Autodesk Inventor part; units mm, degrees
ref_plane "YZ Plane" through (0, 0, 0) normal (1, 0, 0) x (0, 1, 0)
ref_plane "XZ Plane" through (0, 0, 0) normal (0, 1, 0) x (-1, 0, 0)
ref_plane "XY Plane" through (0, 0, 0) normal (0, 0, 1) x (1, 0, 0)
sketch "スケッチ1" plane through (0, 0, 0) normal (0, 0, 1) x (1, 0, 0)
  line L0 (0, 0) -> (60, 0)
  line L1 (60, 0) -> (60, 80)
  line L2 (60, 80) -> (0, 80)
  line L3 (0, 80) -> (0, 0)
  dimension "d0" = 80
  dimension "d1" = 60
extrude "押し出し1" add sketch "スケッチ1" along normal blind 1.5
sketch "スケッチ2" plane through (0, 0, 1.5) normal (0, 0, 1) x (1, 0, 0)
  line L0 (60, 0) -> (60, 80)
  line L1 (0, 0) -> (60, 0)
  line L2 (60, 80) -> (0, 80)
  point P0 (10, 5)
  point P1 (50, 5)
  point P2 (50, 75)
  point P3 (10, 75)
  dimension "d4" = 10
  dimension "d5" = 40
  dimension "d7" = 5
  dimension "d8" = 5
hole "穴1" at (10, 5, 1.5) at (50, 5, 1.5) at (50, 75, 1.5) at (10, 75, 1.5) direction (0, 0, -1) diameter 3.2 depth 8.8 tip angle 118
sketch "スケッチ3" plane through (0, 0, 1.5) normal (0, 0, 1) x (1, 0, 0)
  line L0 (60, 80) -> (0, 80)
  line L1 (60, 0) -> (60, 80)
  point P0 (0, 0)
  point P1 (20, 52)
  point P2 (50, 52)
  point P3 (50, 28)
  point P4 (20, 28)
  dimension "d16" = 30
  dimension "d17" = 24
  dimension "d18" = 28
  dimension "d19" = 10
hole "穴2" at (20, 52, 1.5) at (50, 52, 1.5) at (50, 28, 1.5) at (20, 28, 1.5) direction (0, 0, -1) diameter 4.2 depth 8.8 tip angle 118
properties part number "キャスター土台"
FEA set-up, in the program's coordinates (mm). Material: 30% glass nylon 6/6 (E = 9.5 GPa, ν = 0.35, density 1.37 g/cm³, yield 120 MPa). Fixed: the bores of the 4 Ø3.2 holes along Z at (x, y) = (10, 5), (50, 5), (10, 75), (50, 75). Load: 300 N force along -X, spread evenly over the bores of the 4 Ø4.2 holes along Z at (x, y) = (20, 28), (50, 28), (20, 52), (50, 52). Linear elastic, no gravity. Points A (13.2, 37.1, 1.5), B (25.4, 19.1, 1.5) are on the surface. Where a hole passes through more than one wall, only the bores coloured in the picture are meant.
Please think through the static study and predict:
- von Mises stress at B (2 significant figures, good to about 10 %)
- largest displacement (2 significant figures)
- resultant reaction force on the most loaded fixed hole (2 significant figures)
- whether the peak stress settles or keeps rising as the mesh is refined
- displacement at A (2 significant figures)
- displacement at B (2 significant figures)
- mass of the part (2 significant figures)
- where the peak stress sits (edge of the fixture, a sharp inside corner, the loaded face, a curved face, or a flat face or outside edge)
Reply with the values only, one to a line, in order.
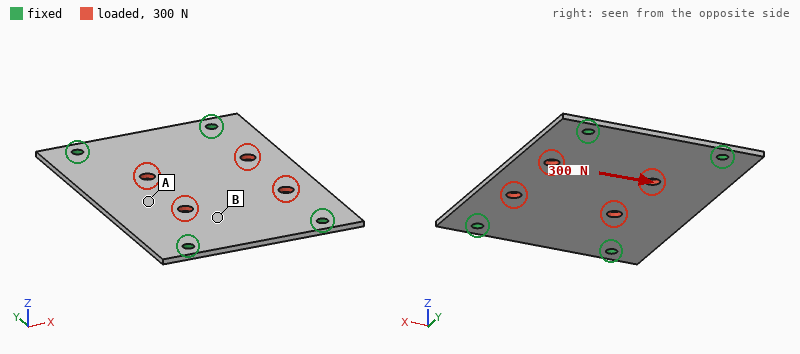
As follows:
4.0 MPa
21 µm
86 N
keeps rising
18 µm
11 µm
9.7 g
edge of the fixture
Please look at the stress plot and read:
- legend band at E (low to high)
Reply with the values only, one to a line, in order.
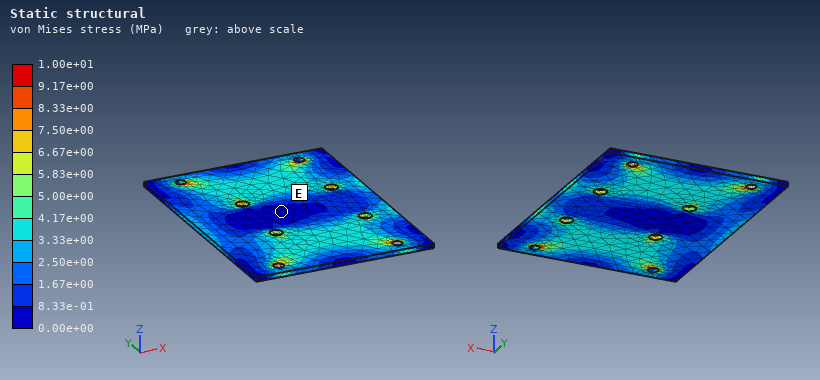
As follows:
0.00e+00 to 8.33e-01 MPa
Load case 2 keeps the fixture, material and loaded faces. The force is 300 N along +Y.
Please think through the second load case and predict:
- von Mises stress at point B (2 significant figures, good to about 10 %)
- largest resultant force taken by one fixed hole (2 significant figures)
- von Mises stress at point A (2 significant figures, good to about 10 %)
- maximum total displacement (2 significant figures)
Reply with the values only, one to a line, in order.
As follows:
1.1 MPa
84 N
1.4 MPa
10 µm
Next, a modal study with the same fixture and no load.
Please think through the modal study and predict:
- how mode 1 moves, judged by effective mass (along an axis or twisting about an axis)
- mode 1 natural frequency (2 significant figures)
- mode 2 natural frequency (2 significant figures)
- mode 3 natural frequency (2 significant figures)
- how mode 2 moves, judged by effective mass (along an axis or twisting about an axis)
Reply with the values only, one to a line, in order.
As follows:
along Z
770 Hz
1000 Hz
1700 Hz
twisting about Y
